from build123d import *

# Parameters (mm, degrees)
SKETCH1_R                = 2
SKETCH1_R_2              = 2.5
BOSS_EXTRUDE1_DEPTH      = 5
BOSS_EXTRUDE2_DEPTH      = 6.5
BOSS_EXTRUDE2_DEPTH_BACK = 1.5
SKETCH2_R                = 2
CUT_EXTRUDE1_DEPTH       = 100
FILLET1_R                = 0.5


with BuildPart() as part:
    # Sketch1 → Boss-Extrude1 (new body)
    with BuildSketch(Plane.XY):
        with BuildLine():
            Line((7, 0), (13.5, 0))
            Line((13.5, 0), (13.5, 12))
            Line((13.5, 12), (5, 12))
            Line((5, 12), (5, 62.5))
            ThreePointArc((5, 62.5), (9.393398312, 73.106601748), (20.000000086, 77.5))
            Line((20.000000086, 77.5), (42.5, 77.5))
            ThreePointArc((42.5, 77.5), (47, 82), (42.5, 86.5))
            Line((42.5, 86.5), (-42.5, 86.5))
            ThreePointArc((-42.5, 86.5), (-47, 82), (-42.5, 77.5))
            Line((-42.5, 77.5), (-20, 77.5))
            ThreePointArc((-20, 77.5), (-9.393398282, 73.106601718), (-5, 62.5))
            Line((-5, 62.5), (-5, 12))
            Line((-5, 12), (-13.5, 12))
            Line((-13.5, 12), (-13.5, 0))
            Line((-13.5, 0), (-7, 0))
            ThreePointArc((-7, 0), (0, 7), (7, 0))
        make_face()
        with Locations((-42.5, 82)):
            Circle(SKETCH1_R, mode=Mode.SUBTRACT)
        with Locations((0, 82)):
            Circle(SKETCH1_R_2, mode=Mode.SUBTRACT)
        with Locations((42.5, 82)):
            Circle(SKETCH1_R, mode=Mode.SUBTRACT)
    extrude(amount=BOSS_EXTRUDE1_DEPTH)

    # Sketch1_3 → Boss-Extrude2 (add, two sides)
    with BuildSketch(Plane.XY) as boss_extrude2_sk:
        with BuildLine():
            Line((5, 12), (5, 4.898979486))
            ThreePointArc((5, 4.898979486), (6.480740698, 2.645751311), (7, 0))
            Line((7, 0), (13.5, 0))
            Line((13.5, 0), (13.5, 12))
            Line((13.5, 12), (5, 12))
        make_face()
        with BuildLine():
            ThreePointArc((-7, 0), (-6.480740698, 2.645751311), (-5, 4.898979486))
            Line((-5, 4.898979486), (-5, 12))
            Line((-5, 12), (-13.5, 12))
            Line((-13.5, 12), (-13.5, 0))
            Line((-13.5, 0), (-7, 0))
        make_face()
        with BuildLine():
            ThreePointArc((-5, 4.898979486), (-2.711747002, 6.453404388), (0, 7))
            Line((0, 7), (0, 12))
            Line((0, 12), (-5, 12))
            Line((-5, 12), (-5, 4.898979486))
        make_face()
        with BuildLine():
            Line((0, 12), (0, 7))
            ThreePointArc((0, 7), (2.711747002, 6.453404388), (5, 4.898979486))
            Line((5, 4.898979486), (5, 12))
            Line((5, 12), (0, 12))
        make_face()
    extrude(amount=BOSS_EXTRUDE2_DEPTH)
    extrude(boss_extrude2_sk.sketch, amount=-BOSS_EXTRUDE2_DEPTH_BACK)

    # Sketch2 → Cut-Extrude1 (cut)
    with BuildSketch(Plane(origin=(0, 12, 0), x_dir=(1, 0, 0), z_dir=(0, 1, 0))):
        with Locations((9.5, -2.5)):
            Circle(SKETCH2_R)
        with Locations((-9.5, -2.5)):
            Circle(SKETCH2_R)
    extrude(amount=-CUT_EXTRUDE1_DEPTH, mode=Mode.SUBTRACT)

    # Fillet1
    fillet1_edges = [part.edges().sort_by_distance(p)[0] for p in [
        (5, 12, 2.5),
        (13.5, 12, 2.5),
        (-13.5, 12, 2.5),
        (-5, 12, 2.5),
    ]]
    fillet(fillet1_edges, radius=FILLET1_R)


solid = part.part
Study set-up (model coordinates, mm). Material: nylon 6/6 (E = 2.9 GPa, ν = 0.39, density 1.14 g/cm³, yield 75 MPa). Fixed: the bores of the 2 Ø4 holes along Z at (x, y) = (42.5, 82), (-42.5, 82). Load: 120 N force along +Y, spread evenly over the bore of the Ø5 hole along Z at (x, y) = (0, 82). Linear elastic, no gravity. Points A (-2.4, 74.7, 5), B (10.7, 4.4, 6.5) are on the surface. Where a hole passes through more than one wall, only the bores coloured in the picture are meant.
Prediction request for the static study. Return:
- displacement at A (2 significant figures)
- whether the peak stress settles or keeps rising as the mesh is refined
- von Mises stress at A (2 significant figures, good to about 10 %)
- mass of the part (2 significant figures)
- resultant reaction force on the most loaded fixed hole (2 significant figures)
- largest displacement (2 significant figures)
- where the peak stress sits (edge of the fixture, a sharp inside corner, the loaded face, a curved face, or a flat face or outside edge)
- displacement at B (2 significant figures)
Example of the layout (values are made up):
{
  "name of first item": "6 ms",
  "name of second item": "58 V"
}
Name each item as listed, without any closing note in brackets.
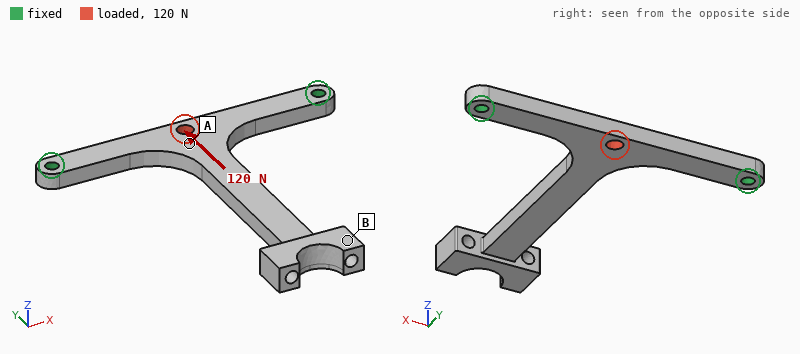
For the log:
{
  "displacement at A": "0.30 mm",
  "whether the peak stress settles or keeps rising as the mesh is refined": "keeps rising",
  "von Mises stress at A": "4.3 MPa",
  "mass of the part": "11 g",
  "resultant reaction force on the most loaded fixed hole": "74 N",
  "largest displacement": "0.31 mm",
  "where the peak stress sits": "edge of the fixture",
  "displacement at B": "0.29 mm"
}
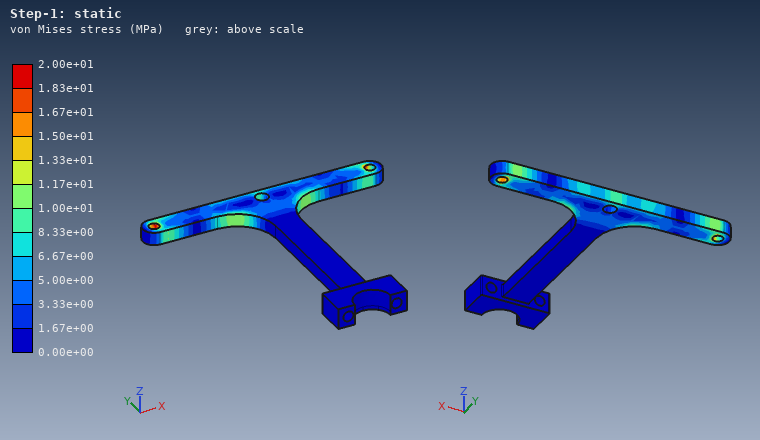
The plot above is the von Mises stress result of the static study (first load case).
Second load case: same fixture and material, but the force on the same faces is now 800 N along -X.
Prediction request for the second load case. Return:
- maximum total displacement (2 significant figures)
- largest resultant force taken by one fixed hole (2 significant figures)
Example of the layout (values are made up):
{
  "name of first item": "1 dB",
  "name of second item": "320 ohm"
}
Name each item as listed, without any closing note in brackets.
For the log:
{
  "maximum total displacement": "0.13 mm",
  "largest resultant force taken by one fixed hole": "400 N"
}
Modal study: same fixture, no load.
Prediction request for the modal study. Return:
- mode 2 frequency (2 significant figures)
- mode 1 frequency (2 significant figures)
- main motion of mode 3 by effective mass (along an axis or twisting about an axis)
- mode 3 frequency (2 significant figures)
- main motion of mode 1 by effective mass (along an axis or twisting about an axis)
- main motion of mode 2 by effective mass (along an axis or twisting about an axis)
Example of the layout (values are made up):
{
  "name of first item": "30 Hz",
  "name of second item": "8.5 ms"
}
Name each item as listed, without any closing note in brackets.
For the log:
{
  "mode 2 frequency": "330 Hz",
  "mode 1 frequency": "110 Hz",
  "main motion of mode 3 by effective mass": "along Z",
  "mode 3 frequency": "720 Hz",
  "main motion of mode 1 by effective mass": "along Z",
  "main motion of mode 2 by effective mass": "along X"
}
